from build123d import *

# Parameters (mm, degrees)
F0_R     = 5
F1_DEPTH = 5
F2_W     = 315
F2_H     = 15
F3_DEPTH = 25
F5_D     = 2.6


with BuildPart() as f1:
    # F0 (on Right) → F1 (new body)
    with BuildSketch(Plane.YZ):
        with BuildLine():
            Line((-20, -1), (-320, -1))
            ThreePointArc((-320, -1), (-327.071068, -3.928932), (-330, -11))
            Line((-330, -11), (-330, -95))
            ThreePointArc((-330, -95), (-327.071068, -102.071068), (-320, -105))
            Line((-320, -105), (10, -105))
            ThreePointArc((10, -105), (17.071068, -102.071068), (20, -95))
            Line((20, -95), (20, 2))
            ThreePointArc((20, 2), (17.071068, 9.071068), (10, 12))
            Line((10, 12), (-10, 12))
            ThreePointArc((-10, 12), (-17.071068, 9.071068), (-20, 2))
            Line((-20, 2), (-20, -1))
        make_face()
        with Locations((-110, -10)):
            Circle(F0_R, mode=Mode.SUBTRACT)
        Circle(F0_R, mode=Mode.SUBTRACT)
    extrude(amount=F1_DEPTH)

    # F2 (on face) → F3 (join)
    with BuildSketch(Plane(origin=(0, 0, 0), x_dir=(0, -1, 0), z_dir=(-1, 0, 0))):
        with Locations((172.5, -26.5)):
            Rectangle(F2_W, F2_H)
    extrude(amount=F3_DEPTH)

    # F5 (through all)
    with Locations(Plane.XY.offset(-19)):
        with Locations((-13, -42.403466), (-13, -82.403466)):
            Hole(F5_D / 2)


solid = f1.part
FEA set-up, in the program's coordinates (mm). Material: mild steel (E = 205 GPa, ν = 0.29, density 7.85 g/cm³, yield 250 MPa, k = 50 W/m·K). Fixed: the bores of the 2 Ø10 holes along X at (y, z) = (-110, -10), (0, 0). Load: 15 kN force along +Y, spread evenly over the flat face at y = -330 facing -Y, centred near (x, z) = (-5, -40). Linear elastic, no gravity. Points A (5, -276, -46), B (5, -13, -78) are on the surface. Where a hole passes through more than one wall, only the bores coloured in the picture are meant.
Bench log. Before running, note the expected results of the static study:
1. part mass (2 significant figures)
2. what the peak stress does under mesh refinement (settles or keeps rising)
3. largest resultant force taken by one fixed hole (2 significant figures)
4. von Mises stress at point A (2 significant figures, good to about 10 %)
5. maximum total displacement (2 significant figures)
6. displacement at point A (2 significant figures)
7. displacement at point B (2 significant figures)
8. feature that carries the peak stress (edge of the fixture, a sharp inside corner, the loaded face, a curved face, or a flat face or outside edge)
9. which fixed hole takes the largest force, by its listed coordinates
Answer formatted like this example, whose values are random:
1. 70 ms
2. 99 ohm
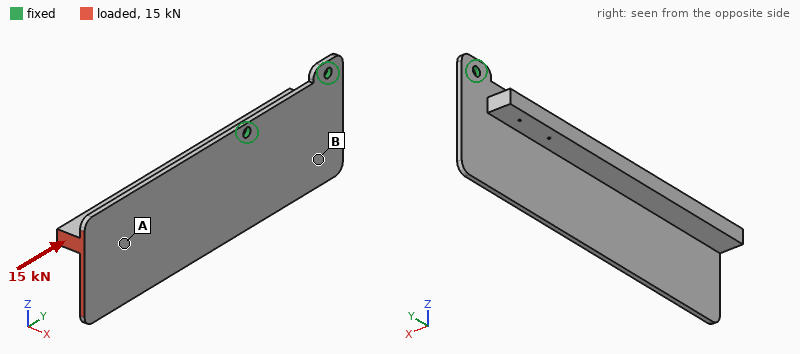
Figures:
1. 2.4 kg
2. keeps rising
3. 11 kN
4. 18 MPa
5. 0.15 mm
6. 0.10 mm
7. 0.048 mm
8. edge of the fixture
9. (-110, -10)
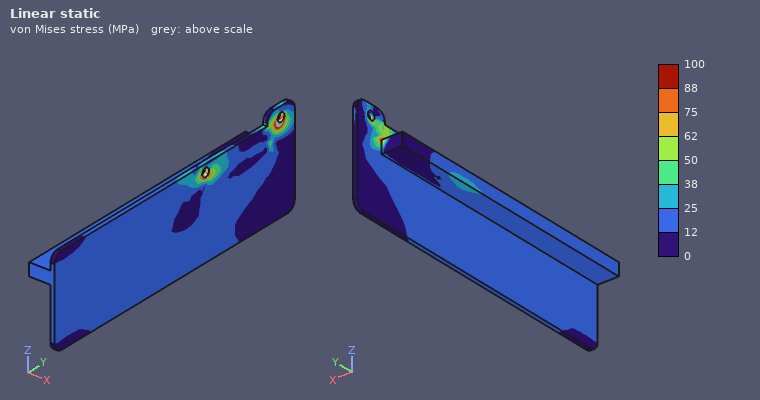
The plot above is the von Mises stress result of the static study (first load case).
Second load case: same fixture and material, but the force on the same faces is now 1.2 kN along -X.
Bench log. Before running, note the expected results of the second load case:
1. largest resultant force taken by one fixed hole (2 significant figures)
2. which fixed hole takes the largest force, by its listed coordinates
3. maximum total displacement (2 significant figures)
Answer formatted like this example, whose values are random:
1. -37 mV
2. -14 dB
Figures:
1. 4.5 kN
2. (-110, -10)
3. 1.0 mm
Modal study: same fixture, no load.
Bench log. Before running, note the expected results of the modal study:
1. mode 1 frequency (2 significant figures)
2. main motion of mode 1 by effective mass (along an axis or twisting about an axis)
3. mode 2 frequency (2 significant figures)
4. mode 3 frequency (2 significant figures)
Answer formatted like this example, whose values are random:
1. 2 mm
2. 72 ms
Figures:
1. 260 Hz
2. along X
3. 370 Hz
4. 690 Hz
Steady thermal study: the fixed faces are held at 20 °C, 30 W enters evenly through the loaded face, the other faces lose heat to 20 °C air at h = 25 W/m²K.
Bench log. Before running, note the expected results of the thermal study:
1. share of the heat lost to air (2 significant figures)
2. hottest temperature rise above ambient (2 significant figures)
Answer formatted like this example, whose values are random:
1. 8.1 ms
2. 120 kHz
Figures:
1. 93 %
2. 59 K
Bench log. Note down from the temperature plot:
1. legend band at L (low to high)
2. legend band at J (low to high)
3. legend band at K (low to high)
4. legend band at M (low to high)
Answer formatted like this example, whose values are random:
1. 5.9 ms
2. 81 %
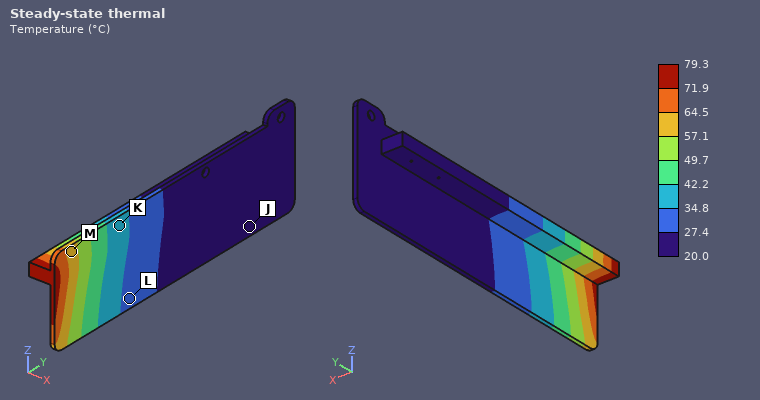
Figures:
1. 27.4 to 34.8 °C
2. 20.0 to 27.4 °C
3. 34.8 to 42.2 °C
4. 57.1 to 64.5 °C
